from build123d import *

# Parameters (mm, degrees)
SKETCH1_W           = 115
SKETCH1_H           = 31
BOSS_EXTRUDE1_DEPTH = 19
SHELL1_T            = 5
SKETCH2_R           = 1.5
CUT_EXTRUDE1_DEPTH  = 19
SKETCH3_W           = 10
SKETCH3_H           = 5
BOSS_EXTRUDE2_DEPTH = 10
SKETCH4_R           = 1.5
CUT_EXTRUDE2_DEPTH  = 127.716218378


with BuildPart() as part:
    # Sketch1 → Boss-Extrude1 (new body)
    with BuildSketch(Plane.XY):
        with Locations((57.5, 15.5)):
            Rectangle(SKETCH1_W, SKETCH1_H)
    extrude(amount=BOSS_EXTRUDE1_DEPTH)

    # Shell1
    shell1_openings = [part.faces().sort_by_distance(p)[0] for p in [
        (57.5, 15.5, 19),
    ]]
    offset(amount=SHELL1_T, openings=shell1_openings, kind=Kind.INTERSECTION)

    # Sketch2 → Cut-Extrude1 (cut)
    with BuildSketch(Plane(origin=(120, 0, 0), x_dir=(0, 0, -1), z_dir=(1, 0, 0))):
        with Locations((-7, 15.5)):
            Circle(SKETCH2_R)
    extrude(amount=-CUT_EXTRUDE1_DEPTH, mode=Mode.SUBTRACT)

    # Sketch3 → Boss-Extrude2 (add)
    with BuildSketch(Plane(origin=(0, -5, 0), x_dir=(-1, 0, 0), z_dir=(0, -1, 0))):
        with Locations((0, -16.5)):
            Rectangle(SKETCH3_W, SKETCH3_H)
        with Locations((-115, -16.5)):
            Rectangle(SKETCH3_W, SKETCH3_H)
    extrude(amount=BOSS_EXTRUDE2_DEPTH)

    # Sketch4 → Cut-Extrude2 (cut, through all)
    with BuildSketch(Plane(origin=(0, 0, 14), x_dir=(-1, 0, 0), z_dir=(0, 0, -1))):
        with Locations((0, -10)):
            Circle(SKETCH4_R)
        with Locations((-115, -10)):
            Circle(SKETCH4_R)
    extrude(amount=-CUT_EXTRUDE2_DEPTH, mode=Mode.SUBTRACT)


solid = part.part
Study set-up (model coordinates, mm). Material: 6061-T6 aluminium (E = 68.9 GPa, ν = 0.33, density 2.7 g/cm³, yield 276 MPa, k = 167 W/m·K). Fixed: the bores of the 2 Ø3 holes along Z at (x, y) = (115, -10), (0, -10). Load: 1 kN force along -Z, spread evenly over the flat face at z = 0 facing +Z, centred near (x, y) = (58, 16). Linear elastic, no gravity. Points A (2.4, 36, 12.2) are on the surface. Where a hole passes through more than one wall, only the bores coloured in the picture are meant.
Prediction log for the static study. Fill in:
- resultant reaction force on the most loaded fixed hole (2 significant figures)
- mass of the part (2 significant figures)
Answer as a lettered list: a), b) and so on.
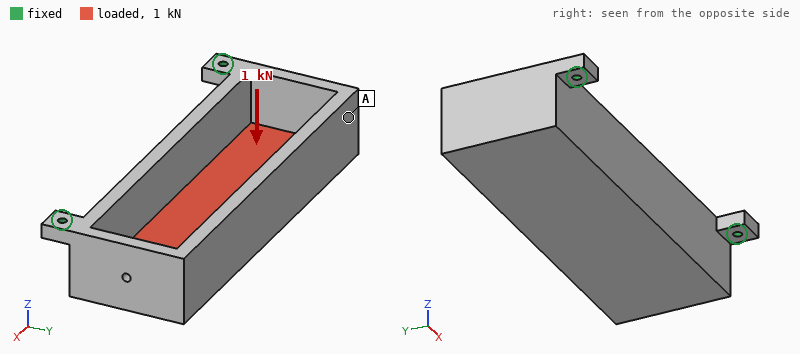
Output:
a) 510 N
b) 150 g
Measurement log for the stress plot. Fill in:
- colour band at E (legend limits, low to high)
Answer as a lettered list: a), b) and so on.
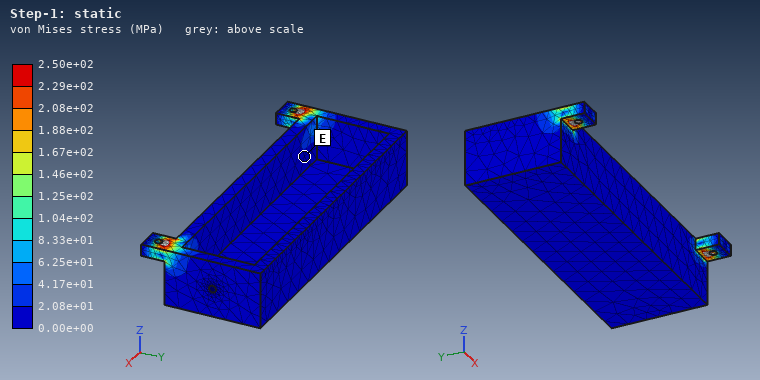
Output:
a) 0.00e+00 to 2.08e+01 MPa
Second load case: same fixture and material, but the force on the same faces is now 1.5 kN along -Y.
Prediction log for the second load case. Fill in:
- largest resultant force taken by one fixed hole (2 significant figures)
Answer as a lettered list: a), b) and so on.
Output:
a) 760 N
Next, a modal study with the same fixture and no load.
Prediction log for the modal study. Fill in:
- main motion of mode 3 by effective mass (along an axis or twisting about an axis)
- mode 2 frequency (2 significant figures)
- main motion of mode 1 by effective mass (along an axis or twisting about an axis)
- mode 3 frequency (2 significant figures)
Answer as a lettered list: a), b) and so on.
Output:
a) along Y
b) 1500 Hz
c) along Z
d) 3300 Hz
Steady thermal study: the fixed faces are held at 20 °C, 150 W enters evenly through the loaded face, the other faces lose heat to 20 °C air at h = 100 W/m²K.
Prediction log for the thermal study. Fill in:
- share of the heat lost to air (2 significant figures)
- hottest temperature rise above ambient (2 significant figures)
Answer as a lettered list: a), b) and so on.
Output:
a) 62 %
b) 60 K
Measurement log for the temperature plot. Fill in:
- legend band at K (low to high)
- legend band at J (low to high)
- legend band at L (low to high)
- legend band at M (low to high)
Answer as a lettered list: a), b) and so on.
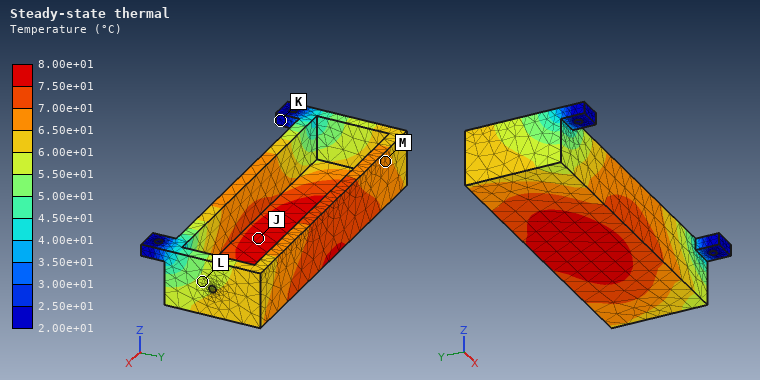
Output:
a) 2.00e+01 to 2.50e+01 °C
b) 7.50e+01 to 8.00e+01 °C
c) 5.50e+01 to 6.00e+01 °C
d) 6.50e+01 to 7.00e+01 °C
